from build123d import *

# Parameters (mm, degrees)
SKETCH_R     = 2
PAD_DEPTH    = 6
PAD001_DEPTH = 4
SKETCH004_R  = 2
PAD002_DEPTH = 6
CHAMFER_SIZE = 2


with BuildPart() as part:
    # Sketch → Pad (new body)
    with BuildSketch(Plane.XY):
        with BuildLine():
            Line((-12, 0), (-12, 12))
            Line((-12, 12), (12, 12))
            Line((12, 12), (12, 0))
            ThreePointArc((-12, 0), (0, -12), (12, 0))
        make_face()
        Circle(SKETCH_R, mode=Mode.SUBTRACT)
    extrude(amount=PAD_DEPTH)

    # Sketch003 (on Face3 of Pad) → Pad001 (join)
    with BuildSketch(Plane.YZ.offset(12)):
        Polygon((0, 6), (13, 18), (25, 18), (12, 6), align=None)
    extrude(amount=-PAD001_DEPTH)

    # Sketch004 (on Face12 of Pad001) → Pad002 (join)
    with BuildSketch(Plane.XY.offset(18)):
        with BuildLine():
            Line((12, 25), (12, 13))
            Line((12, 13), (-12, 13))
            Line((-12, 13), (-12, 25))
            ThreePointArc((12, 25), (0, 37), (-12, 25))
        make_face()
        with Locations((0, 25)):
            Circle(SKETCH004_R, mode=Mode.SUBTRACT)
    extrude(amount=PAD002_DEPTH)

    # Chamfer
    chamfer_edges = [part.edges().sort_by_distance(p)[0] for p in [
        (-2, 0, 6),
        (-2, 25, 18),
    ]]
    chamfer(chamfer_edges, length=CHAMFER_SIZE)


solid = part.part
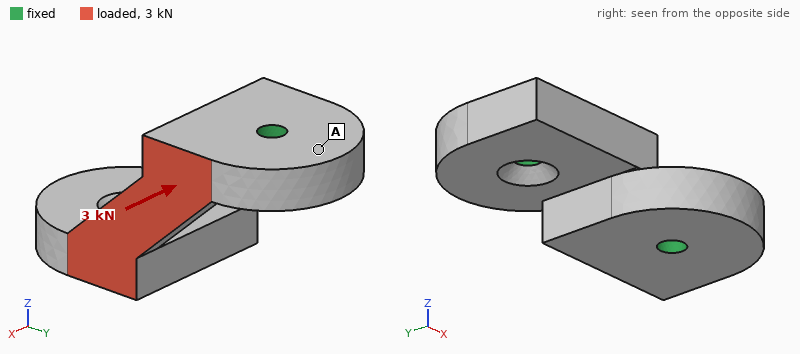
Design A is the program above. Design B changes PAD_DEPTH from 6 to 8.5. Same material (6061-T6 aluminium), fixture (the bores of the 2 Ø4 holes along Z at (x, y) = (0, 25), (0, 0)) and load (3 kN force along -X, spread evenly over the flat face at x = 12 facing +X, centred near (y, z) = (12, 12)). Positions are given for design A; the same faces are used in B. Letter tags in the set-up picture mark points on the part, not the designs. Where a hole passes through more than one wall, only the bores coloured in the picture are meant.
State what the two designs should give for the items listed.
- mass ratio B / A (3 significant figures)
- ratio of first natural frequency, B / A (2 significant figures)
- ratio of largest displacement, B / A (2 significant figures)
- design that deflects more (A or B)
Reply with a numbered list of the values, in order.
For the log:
1. 1.18
2. 1.1
3. 0.77
4. A
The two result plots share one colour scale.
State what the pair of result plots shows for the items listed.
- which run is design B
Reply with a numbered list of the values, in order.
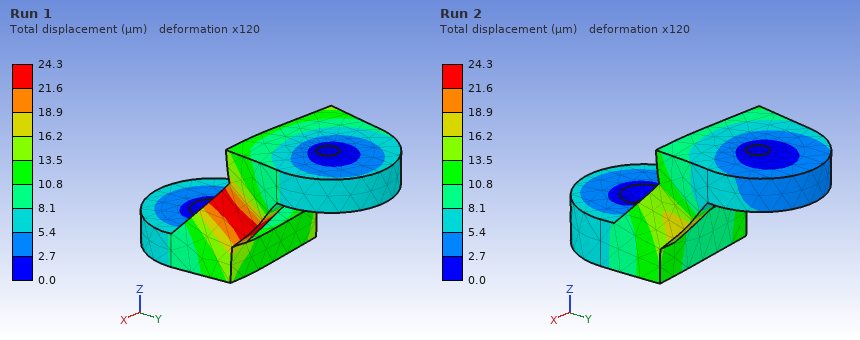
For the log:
1. Run 2
